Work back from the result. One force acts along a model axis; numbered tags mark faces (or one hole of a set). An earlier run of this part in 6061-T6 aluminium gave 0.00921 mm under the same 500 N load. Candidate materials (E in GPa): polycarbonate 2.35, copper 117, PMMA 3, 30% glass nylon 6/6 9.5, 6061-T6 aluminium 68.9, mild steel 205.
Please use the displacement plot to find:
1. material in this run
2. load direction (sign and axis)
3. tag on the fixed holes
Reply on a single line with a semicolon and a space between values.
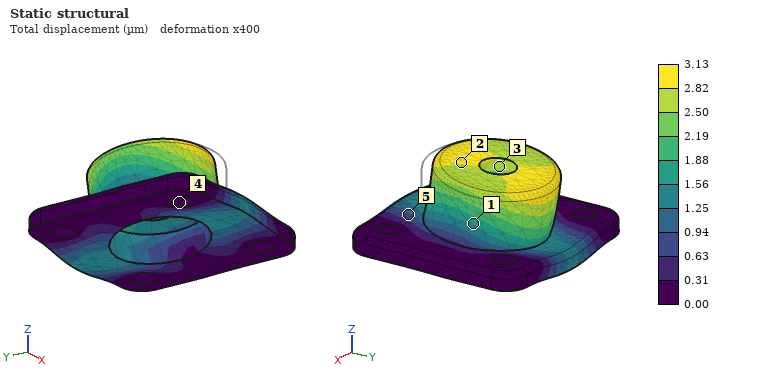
mild steel; +Y; 4
